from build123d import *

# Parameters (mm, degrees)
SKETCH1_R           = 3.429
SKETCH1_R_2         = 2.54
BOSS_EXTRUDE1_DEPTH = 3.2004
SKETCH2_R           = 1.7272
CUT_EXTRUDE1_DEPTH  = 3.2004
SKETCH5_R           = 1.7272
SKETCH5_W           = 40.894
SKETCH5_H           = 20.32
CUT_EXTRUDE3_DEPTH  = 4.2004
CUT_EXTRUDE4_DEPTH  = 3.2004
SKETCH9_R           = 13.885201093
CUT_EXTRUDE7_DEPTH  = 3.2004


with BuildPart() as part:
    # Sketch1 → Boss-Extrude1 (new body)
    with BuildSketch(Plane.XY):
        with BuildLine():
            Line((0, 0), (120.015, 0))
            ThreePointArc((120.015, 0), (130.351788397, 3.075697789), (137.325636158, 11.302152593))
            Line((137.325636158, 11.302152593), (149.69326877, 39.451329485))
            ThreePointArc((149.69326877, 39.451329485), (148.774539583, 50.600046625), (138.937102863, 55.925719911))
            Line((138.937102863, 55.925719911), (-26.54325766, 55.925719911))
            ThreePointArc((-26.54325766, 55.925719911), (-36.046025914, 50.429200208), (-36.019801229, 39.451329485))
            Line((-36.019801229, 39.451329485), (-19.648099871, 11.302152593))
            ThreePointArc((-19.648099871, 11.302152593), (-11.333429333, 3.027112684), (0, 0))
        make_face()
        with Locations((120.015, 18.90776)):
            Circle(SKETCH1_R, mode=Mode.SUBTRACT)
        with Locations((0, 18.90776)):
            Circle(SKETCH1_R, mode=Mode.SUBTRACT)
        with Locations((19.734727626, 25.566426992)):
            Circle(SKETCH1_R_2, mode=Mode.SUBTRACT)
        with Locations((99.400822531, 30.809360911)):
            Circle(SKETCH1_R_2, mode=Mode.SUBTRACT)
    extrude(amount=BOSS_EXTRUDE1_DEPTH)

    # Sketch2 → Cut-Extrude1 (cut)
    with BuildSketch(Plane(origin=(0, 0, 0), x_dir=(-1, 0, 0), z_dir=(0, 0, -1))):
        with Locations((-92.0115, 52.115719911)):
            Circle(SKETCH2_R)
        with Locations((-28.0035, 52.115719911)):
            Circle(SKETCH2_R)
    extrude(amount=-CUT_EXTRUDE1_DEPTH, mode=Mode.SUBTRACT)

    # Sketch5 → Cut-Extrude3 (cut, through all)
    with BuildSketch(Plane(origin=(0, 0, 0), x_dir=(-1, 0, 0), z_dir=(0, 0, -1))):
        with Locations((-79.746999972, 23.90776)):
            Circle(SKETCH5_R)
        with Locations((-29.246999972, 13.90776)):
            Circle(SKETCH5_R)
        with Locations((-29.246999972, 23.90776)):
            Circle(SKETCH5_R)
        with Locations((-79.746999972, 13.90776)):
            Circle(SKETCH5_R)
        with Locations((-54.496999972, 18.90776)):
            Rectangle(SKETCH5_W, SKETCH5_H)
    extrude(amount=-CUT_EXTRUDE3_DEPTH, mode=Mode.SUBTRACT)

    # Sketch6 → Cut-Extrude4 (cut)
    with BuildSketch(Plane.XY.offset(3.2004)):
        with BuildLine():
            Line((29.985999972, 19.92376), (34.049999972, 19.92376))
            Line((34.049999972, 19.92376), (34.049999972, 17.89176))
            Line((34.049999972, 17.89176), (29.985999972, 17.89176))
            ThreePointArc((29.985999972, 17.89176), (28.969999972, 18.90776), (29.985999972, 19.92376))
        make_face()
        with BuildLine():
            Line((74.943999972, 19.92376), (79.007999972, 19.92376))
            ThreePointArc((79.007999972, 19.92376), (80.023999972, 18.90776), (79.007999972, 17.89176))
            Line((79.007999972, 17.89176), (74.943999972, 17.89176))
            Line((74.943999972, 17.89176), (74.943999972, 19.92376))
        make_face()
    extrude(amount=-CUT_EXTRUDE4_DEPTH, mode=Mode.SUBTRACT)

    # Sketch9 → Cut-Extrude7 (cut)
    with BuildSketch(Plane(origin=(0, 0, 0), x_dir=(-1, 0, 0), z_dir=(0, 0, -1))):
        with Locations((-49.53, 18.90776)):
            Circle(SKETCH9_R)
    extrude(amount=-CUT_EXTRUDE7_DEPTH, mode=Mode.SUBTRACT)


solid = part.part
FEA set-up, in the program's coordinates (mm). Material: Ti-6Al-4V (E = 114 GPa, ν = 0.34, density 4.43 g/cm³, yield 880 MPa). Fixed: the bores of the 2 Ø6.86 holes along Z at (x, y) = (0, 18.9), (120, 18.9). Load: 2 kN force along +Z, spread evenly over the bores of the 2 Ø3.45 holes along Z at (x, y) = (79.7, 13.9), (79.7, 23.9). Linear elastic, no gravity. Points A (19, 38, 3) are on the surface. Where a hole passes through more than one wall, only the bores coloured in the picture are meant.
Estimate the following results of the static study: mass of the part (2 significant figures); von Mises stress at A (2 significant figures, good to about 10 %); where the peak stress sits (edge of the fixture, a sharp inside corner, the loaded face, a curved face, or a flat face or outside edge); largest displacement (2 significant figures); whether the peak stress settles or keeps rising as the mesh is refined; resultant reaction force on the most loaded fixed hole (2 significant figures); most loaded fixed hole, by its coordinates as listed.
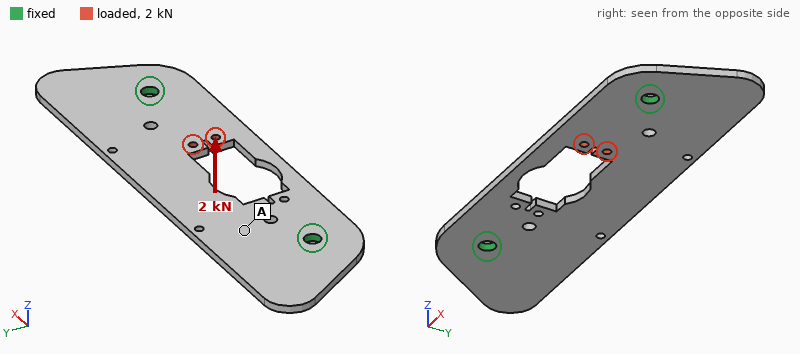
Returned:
120 g
95 MPa
edge of the fixture
1.4 mm
keeps rising
1.5 kN
(120, 18.9)
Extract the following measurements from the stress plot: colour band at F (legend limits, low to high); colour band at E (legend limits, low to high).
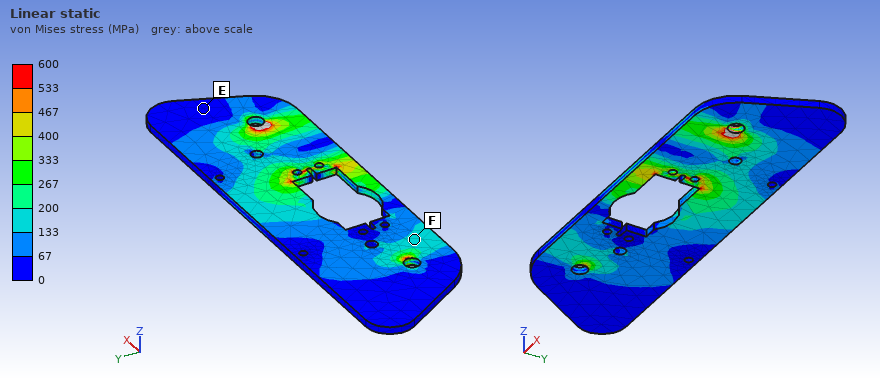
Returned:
133 to 200 MPa
0 to 67 MPa
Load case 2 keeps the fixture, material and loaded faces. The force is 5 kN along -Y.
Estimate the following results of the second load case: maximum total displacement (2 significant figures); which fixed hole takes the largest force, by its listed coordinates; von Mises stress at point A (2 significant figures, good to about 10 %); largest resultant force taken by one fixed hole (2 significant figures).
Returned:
85 µm
(120, 18.9)
24 MPa
3.8 kN
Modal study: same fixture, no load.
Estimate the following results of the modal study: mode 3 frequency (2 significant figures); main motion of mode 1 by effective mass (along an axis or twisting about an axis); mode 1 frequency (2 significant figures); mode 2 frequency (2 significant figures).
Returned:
1700 Hz
along Z
1000 Hz
1500 Hz
